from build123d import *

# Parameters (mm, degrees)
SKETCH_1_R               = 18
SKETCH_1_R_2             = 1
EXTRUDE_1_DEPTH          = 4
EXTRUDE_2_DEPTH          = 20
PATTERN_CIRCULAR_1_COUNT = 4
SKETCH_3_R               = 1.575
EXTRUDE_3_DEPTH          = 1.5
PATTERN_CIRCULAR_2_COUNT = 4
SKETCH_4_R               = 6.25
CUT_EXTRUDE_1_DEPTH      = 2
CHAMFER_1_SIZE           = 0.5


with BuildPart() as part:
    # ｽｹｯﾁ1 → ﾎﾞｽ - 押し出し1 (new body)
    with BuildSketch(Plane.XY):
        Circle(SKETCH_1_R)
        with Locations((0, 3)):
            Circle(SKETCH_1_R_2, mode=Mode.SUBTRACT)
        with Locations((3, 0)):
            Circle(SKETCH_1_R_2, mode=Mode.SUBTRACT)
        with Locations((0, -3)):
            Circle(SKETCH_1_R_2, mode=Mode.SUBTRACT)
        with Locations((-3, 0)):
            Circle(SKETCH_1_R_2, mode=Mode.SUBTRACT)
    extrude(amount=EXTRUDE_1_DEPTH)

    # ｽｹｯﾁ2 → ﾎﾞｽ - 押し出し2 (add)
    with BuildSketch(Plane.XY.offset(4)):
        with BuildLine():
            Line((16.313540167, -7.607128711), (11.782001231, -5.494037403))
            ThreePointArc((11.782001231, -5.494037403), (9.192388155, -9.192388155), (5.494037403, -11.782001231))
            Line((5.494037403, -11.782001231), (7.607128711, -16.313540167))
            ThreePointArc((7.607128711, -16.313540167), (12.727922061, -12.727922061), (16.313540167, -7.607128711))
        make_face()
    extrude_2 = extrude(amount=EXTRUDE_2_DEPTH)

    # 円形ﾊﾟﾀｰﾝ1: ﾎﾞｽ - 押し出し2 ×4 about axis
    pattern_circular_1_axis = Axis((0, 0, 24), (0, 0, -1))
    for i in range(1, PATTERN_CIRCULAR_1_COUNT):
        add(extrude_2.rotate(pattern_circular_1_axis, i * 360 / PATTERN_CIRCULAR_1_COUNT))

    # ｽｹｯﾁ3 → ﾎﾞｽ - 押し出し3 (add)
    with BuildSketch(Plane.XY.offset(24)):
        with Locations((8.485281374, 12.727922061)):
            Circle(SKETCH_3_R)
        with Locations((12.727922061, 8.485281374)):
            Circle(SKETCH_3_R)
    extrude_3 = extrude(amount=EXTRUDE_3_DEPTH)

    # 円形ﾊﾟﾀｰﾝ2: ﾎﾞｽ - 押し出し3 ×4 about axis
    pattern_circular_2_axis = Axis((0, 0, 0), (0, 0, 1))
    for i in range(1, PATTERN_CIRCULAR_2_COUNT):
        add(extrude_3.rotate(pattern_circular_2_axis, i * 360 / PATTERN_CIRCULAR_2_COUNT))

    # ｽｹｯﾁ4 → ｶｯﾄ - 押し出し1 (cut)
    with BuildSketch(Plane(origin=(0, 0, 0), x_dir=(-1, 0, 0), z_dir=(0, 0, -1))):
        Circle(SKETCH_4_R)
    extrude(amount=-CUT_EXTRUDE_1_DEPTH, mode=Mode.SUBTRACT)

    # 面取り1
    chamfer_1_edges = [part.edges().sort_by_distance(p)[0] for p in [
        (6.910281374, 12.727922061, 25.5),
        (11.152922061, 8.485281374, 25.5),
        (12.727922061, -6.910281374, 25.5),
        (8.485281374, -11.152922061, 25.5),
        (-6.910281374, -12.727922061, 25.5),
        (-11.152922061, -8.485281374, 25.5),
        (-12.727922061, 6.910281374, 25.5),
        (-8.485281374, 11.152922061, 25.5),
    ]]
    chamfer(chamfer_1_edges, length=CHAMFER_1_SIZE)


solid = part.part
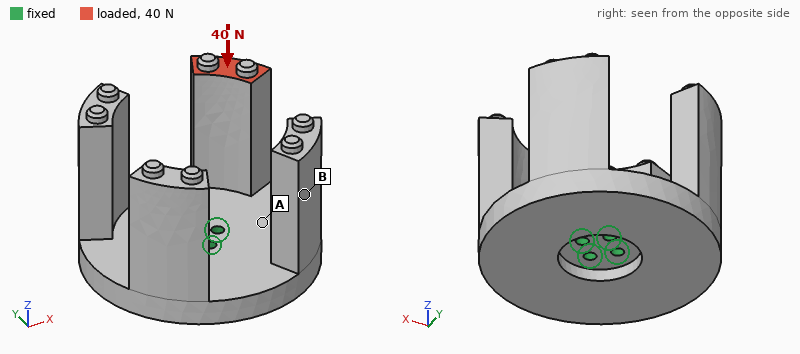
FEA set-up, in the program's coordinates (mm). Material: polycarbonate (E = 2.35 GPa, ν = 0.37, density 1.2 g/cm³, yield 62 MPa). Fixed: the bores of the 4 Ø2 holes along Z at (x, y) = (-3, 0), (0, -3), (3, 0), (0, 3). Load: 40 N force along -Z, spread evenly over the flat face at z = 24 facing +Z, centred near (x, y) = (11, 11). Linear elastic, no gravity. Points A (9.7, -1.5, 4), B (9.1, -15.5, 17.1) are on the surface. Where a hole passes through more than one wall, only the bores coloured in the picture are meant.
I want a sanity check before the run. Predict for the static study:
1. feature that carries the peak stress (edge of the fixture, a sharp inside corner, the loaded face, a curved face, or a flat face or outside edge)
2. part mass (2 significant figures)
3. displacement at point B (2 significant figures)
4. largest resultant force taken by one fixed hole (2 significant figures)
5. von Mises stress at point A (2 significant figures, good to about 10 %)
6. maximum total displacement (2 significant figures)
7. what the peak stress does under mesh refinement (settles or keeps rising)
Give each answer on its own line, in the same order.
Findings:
edge of the fixture
9.9 g
0.16 mm
47 N
5.2 MPa
0.60 mm
keeps rising
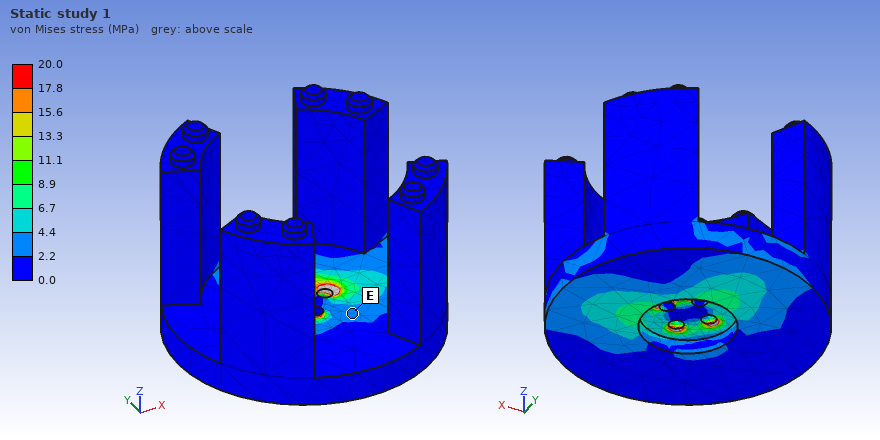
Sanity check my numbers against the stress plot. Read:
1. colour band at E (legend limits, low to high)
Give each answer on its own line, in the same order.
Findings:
2.2 to 4.4 MPa
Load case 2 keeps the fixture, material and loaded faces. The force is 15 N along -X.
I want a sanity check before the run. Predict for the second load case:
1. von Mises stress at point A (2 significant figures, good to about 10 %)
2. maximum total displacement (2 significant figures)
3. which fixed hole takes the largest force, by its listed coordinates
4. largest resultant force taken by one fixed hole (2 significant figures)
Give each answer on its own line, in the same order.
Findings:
3.1 MPa
0.56 mm
(3, 0)
33 N
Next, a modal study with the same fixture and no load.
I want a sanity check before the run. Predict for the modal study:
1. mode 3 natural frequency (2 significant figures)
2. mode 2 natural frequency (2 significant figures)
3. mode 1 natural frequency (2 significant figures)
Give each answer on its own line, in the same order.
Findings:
1200 Hz
750 Hz
750 Hz
